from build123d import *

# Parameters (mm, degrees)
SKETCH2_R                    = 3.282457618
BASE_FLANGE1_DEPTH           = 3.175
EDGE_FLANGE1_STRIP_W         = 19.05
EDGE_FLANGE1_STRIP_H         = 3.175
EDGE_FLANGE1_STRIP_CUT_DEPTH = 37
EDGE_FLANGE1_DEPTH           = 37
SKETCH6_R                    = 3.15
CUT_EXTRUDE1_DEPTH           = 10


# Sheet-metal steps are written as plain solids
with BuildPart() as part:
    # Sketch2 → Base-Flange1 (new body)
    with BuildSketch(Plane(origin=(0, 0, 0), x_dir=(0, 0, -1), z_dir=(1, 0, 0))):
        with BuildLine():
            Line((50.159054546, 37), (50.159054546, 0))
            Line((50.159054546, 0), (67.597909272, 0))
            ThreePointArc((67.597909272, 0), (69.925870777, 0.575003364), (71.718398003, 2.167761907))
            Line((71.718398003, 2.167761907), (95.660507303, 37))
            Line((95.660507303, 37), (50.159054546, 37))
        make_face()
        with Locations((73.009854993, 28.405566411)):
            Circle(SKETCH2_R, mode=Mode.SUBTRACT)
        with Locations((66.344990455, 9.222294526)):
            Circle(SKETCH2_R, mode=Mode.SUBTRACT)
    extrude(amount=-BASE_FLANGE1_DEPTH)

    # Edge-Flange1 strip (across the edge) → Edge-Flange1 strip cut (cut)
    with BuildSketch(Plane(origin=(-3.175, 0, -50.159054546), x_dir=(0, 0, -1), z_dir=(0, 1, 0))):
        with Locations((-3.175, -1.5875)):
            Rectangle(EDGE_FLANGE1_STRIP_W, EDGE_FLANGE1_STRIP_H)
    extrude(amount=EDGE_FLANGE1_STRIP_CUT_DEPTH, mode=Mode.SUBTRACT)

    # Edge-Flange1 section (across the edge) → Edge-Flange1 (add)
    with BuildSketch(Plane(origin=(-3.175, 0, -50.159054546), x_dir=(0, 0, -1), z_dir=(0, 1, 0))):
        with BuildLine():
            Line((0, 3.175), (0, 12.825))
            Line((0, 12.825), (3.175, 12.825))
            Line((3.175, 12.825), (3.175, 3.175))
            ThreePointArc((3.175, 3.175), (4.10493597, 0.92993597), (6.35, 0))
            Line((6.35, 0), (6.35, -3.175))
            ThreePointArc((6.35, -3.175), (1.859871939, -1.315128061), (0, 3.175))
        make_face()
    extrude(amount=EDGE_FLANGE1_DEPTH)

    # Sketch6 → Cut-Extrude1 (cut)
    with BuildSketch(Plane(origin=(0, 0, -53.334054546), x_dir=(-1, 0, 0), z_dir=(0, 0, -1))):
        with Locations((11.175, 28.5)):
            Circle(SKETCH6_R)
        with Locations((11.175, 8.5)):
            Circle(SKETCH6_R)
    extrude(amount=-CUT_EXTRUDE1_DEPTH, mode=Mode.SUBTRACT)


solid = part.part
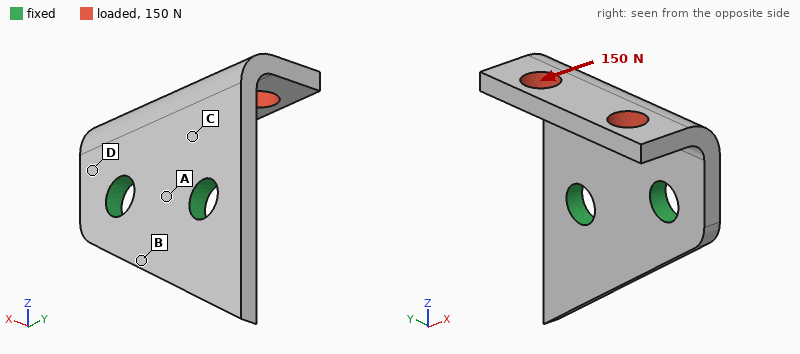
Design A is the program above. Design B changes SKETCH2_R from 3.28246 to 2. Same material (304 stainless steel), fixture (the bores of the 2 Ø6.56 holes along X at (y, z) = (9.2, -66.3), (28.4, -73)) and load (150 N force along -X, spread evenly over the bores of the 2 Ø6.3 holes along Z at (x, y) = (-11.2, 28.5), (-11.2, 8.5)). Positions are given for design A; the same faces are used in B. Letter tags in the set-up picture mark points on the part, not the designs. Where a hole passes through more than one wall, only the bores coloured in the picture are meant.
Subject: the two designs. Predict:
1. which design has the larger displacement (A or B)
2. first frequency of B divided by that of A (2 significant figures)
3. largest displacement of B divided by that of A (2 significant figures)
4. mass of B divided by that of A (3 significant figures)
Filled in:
B
0.89
1.3
1.03
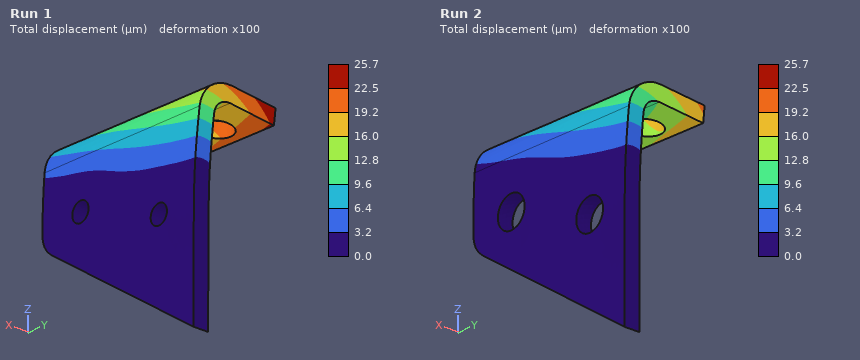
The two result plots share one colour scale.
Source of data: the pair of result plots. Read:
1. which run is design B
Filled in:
Run 1
